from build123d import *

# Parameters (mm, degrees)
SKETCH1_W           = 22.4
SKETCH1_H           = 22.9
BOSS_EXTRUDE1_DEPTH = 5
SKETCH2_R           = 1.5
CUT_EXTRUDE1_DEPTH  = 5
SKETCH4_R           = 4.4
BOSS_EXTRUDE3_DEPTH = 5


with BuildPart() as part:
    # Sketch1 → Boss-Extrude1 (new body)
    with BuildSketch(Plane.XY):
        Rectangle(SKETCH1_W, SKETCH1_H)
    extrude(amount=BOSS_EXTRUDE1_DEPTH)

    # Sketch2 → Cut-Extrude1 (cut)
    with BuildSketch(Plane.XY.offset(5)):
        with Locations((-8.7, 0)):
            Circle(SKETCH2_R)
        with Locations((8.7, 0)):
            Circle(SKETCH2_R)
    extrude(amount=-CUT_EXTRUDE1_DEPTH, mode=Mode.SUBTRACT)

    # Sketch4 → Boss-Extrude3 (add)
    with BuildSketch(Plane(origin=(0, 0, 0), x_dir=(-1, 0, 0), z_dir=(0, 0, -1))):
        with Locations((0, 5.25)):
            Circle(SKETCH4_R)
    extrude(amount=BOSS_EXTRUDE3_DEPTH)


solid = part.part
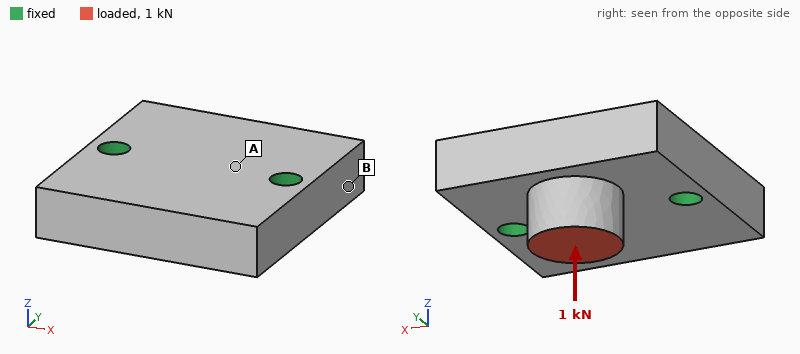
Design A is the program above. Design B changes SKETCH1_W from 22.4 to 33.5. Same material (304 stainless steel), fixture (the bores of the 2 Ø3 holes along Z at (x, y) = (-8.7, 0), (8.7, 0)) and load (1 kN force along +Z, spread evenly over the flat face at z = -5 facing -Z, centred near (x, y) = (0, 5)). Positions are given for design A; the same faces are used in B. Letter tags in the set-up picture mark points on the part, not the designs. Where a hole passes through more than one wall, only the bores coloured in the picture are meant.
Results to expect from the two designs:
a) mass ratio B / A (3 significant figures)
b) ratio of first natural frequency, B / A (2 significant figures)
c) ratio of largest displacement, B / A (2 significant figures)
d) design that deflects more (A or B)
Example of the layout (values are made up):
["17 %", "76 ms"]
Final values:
["1.45", "0.96", "0.88", "A"]
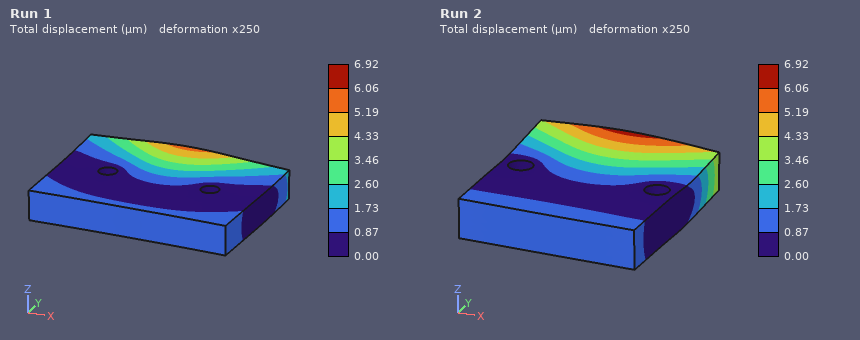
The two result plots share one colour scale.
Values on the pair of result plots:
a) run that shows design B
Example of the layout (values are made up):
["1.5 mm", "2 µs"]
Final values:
["Run 1"]
